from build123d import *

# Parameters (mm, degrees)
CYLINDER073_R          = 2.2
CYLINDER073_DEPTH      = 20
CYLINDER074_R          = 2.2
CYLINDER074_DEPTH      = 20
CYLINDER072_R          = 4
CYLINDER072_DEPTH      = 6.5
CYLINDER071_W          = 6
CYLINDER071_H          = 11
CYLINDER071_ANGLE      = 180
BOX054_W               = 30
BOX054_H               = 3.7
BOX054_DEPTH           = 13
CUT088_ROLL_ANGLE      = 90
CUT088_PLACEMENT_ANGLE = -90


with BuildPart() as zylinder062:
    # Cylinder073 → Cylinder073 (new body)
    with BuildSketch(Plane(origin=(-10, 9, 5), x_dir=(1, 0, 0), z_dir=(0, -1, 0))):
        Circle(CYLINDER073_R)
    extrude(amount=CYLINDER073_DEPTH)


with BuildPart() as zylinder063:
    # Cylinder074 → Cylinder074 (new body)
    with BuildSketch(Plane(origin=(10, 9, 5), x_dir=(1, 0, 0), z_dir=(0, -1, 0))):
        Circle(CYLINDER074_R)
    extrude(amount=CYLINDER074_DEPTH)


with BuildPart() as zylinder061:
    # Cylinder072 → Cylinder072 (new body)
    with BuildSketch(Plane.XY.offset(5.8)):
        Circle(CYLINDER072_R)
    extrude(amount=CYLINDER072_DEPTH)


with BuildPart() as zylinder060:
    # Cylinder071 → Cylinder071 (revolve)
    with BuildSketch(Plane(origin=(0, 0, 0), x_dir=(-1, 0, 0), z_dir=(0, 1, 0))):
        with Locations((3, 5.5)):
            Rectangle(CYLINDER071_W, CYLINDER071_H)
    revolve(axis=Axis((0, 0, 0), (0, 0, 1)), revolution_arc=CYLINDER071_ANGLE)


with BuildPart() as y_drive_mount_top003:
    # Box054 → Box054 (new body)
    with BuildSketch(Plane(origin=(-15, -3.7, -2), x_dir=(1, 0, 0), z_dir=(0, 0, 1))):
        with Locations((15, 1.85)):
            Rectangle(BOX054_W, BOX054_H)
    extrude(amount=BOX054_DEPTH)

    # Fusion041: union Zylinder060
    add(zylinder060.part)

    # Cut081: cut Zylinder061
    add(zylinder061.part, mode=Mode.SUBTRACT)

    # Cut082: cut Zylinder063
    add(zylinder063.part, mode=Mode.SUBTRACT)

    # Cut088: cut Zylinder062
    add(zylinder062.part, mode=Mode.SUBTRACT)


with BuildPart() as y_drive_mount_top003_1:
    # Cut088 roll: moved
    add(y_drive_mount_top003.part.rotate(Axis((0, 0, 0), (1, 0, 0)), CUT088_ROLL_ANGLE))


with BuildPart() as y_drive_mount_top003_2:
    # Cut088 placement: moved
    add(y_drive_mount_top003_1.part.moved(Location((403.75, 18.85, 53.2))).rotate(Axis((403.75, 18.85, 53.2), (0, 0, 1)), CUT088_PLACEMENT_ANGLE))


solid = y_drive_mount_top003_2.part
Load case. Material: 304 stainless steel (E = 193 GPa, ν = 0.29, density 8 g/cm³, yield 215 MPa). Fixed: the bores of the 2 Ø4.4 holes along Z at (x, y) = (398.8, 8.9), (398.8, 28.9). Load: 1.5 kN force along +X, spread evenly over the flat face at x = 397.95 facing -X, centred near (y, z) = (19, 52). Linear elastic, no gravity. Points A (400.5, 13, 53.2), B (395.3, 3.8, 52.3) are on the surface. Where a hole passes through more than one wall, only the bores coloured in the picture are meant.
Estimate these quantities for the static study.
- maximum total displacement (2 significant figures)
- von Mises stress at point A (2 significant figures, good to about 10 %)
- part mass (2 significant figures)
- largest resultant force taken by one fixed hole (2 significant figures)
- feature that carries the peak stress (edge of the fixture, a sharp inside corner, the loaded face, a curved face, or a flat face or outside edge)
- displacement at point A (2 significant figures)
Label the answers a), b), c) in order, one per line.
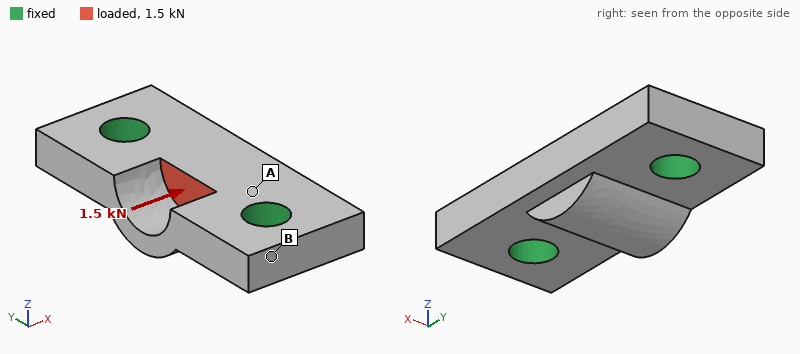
a) 4.1 µm
b) 47 MPa
c) 11 g
d) 790 N
e) edge of the fixture
f) 1.2 µm
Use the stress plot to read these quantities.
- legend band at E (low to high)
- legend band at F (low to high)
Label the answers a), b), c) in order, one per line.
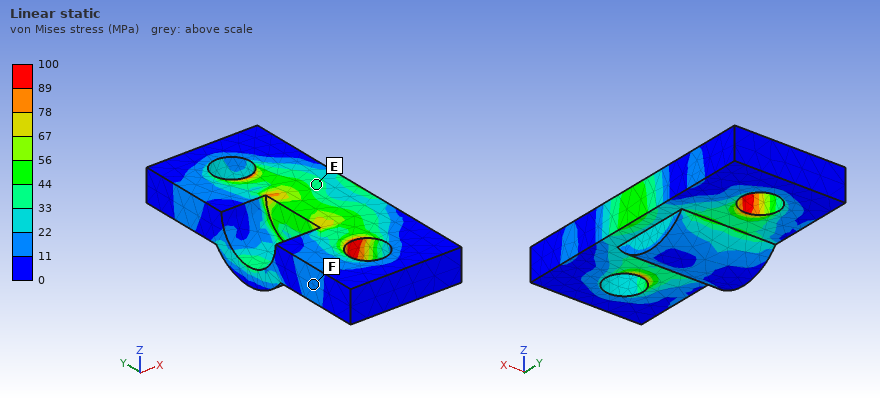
a) 33 to 44 MPa
b) 11 to 22 MPa
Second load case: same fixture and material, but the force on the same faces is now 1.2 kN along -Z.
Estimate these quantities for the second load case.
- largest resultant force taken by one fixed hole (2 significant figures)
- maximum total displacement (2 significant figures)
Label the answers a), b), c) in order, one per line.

a) 660 N
b) 6.4 µm
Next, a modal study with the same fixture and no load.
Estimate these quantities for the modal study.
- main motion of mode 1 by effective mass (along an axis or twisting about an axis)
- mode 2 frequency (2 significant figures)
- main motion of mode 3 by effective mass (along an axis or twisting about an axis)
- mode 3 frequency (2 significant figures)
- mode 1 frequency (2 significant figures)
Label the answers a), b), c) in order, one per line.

a) along Z
b) 50 kHz
c) along X
d) 64 kHz
e) 40 kHz
